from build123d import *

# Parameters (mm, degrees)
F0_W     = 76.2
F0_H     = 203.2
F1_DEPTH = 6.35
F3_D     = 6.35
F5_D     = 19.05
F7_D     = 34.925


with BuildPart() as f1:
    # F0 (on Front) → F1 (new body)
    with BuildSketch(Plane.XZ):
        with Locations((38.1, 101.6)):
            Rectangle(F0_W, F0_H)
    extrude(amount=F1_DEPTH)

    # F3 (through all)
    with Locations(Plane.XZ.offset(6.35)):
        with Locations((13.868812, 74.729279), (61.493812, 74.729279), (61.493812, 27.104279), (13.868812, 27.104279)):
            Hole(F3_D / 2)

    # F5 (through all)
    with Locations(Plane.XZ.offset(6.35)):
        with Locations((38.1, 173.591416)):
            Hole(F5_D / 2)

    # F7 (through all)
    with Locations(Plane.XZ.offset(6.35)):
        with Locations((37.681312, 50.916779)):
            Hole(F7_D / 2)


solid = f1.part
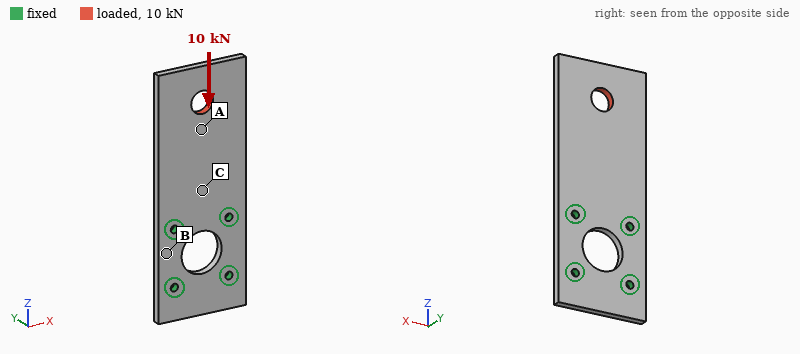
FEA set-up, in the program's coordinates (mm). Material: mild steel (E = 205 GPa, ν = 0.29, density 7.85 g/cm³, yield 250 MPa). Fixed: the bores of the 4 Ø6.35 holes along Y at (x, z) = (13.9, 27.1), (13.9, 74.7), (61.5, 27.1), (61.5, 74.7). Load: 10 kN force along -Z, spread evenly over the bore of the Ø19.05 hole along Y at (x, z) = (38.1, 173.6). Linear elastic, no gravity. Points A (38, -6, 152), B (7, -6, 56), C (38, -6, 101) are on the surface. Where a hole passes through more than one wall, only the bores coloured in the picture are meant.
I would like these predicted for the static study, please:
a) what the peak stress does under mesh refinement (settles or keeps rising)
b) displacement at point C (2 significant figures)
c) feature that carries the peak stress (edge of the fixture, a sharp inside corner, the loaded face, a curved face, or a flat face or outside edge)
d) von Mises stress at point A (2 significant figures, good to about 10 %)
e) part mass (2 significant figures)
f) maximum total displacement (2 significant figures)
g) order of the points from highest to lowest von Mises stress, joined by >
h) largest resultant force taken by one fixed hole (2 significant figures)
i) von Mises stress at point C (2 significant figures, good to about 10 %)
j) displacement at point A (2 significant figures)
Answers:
keeps rising
3.9 µm
edge of the fixture
28 MPa
700 g
16 µm
A > C > B
4.7 kN
17 MPa
9.2 µm
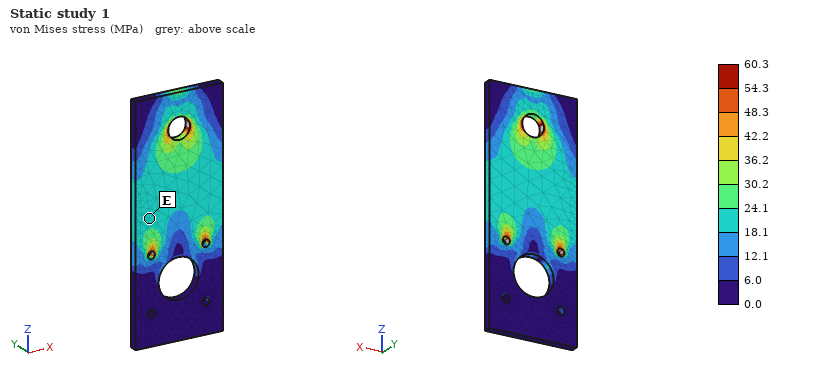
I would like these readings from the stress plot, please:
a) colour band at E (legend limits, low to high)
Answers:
18.1 to 24.1 MPa
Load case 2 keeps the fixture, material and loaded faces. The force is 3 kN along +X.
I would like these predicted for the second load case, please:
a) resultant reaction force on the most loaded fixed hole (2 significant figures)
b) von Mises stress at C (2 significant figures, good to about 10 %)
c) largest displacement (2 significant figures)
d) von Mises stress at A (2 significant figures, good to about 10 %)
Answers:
5.3 kN
17 MPa
46 µm
19 MPa
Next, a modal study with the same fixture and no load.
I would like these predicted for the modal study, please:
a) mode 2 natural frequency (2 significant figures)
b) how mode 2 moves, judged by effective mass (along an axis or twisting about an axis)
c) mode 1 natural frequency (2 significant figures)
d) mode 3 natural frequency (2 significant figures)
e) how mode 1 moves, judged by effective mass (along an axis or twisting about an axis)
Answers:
1200 Hz
twisting about Z
320 Hz
1900 Hz
along Y
